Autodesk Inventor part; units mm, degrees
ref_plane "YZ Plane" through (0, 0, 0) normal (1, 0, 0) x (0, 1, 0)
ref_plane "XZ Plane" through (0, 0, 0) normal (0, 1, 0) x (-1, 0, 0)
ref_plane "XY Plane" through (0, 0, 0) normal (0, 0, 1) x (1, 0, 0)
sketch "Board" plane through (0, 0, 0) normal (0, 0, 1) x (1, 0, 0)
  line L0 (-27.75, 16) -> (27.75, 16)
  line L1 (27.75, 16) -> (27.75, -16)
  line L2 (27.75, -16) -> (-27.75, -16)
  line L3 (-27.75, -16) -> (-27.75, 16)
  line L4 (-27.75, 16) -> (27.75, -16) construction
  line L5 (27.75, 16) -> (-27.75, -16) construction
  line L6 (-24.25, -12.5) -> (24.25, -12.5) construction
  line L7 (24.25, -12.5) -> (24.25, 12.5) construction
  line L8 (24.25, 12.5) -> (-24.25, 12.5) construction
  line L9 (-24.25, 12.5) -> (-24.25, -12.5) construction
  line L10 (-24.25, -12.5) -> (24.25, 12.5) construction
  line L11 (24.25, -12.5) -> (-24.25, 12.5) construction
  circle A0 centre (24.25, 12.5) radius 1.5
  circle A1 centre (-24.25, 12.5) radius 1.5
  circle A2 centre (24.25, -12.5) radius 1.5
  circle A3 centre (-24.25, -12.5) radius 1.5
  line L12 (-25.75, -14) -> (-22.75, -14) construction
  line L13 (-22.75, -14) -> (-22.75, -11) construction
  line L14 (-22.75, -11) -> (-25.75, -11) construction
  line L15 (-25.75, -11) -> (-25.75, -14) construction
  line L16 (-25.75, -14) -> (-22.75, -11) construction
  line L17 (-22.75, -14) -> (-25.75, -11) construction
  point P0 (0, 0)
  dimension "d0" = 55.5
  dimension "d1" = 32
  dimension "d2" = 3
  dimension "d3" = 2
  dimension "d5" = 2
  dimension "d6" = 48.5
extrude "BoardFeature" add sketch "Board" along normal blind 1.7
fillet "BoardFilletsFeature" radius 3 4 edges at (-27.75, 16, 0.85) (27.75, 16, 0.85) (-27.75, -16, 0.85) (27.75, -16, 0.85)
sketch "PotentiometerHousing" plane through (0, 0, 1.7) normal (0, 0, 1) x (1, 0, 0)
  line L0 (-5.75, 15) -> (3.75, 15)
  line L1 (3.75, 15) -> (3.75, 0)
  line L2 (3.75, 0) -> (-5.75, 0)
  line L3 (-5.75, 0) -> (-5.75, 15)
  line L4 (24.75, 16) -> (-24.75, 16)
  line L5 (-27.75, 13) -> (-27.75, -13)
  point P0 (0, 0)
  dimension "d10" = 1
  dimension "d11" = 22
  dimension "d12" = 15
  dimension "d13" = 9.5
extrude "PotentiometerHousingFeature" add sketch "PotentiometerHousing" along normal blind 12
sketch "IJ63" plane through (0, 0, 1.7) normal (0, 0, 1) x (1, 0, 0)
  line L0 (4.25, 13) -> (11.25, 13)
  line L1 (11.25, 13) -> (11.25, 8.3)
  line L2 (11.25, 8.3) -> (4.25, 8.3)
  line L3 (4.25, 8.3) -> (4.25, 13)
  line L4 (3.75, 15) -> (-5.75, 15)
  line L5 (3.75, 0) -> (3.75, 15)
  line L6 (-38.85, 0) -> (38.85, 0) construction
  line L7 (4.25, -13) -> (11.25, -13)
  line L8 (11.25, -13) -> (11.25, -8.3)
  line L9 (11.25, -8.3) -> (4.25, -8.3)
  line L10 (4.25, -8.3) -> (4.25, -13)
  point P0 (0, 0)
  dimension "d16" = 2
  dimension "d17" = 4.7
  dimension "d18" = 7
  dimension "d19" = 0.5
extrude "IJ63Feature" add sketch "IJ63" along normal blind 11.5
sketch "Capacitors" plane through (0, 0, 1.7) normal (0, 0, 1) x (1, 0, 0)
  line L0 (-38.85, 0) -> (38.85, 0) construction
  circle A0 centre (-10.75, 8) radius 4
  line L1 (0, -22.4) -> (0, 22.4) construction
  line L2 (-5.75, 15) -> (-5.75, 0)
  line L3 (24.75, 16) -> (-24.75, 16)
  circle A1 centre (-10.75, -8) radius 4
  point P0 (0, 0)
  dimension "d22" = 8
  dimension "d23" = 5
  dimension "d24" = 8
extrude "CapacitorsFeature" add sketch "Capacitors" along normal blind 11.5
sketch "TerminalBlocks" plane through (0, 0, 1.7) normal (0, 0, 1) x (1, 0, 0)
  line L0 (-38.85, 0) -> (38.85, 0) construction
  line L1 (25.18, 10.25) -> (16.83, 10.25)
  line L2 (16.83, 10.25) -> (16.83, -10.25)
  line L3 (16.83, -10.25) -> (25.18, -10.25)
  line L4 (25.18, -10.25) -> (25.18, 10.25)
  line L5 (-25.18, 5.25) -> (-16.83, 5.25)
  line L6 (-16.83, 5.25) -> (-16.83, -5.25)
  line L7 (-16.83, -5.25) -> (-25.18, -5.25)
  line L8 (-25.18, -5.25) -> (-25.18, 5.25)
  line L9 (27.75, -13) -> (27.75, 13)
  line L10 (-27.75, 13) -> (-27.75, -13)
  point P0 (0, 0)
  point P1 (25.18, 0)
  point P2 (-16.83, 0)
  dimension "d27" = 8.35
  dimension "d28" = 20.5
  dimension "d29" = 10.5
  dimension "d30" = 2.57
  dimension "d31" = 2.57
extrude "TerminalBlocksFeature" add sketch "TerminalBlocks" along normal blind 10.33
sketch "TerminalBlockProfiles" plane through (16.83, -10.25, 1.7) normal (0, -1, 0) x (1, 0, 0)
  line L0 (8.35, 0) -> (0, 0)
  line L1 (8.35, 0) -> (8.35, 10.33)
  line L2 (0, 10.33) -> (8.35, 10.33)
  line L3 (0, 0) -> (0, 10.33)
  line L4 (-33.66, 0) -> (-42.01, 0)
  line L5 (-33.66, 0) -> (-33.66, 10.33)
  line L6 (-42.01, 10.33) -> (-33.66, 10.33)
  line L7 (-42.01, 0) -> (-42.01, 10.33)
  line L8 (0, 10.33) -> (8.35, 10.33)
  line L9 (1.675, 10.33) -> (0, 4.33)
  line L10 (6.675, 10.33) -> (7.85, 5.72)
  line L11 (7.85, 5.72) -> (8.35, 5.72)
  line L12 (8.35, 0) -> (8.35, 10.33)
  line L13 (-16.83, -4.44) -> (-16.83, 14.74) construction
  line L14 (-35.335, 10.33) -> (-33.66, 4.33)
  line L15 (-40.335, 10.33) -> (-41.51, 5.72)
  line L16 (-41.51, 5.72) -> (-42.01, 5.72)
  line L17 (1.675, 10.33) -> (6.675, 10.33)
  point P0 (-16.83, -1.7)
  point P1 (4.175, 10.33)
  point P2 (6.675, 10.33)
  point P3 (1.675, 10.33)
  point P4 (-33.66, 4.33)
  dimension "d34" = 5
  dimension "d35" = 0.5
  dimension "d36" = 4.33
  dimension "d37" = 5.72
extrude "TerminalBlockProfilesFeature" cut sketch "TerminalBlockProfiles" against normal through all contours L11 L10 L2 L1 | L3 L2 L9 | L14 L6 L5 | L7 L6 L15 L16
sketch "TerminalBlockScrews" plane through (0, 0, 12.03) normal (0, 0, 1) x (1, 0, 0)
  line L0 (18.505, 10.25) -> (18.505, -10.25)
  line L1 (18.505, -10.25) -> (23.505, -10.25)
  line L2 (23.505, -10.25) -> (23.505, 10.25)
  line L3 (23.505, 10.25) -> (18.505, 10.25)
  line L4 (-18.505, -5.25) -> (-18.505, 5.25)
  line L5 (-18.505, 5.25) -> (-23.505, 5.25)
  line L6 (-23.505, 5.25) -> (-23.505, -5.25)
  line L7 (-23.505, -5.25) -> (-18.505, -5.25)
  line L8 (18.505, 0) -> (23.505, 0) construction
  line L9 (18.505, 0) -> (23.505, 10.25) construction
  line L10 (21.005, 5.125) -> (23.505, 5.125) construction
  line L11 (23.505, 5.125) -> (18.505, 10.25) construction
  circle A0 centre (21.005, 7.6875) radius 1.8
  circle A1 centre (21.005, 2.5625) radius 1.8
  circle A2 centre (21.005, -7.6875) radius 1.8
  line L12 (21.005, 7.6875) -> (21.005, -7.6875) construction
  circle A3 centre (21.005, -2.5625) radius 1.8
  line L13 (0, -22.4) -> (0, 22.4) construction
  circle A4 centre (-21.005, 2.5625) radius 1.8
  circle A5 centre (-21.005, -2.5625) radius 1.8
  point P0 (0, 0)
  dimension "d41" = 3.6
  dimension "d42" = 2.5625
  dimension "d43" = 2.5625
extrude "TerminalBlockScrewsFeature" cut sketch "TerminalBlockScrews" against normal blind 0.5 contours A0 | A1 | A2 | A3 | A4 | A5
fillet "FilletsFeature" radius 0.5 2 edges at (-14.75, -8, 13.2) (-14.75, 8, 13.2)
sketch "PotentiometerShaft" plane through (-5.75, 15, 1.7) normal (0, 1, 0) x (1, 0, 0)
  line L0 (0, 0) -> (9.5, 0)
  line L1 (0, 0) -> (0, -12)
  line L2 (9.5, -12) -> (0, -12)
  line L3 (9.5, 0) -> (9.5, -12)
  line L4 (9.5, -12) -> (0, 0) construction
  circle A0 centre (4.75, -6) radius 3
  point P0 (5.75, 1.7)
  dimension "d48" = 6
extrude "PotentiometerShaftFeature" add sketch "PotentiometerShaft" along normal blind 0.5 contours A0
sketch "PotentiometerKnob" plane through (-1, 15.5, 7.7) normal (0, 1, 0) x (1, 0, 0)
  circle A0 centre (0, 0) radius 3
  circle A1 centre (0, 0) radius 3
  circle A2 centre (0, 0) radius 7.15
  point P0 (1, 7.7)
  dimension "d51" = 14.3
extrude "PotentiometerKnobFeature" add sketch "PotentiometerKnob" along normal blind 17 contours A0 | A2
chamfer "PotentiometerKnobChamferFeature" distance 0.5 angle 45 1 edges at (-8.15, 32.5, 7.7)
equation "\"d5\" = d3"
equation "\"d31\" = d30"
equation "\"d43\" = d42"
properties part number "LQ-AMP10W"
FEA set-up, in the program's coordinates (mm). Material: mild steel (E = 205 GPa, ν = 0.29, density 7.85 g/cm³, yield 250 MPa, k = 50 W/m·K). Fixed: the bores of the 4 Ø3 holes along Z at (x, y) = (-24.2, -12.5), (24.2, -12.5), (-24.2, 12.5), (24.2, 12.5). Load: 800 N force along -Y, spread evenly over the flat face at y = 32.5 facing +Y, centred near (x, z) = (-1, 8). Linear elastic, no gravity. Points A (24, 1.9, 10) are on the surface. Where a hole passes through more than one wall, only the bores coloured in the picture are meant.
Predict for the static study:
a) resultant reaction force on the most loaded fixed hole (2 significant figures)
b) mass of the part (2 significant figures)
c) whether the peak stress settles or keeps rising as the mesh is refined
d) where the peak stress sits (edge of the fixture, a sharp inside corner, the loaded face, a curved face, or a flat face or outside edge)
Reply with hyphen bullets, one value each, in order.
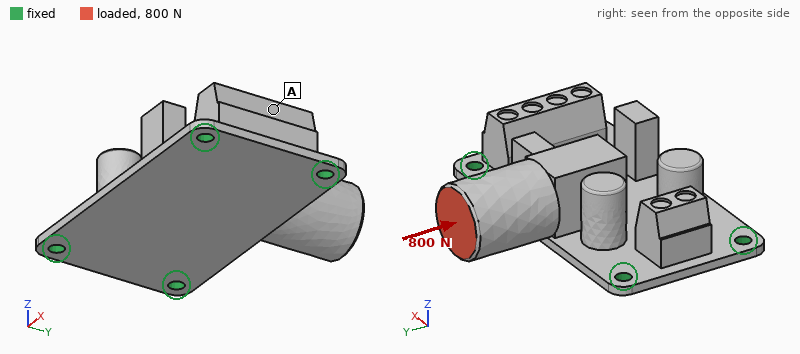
- 320 N
- 91 g
- keeps rising
- edge of the fixture
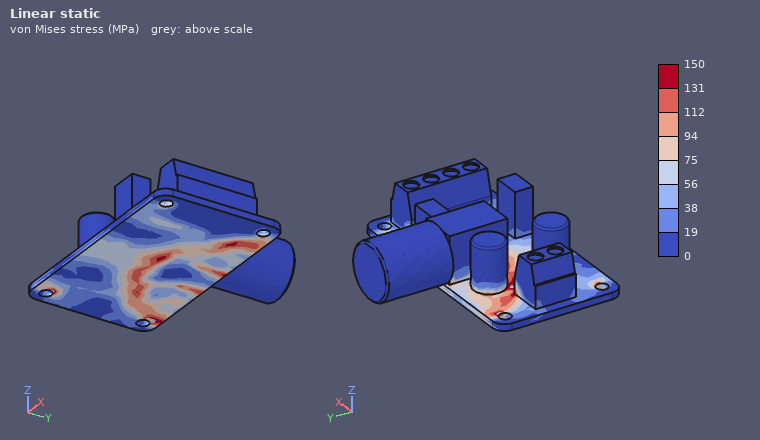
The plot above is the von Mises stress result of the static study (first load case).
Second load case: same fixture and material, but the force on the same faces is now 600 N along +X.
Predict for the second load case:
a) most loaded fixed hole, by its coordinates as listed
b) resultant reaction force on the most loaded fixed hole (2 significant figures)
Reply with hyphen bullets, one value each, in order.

- (-24.2, 12.5)
- 290 N
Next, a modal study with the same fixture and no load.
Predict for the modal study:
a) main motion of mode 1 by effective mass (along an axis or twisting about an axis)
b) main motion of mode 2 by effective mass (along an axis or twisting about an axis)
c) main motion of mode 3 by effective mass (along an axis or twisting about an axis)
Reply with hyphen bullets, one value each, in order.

- along Z
- along Z
- along X
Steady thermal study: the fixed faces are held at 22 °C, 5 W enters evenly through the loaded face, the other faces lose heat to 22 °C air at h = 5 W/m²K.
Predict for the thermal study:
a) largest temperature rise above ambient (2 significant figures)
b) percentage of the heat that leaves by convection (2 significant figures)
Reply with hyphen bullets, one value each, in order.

- 43 K
- 10 %
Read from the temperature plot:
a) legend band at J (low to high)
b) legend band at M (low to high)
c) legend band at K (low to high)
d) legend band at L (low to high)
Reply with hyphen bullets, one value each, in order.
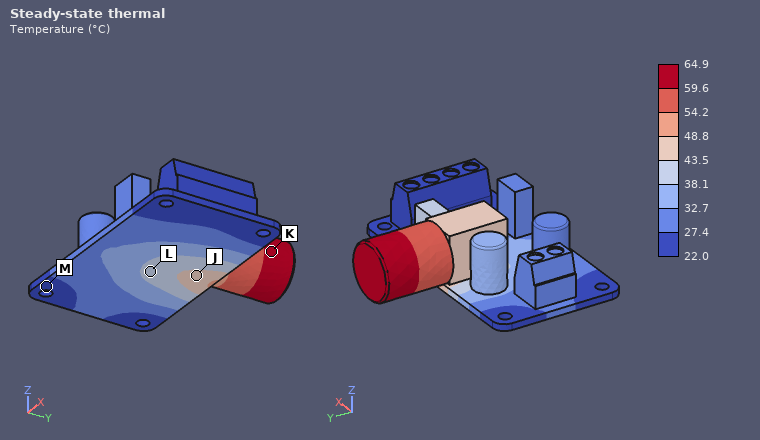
- 43.5 to 48.8 °C
- 22.0 to 27.4 °C
- 59.6 to 64.9 °C
- 38.1 to 43.5 °C
